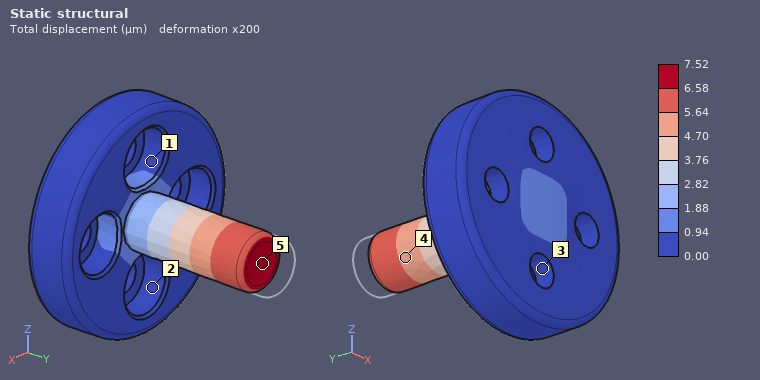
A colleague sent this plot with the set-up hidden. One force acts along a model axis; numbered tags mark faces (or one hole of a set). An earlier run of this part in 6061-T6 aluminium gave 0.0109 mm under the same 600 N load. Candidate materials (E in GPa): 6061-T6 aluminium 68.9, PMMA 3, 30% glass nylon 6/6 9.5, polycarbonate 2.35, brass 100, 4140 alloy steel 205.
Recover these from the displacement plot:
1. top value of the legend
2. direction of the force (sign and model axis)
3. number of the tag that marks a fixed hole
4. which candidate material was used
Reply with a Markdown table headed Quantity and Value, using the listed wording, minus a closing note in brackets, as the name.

| Quantity | Value |
|---|---|
| top value of the legend | 7.52 µm |
| direction of the force | -Y |
| number of the tag that marks a fixed hole | 3 |
| which candidate material was used | brass |
